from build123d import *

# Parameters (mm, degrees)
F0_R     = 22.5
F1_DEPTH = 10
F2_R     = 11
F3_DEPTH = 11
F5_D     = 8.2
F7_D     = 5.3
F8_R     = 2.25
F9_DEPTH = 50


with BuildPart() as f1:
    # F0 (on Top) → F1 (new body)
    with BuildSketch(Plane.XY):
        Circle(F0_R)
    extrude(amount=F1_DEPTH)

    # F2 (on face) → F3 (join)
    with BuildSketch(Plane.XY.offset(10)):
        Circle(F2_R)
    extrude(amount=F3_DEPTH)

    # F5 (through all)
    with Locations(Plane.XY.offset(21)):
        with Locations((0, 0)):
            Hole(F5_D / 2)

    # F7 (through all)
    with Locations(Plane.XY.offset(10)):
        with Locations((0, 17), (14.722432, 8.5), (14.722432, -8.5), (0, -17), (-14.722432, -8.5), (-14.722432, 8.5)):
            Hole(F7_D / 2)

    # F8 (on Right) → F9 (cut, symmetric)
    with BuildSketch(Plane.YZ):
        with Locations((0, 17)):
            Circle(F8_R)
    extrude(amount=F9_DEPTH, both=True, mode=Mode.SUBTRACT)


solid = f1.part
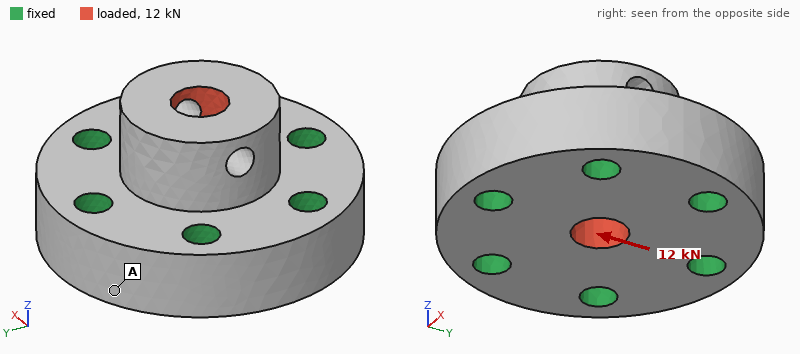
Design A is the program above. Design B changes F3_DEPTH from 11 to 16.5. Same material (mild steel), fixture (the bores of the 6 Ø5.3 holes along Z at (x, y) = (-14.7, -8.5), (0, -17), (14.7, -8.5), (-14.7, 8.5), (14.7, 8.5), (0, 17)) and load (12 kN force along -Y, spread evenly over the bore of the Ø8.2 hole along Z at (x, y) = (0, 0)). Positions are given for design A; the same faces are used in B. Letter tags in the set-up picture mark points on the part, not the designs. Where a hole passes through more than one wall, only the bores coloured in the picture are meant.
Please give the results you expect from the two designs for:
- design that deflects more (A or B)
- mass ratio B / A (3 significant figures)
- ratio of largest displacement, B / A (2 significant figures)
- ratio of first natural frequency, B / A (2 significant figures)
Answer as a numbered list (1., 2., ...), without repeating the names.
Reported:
1. B
2. 1.10
3. 1.8
4. 0.63
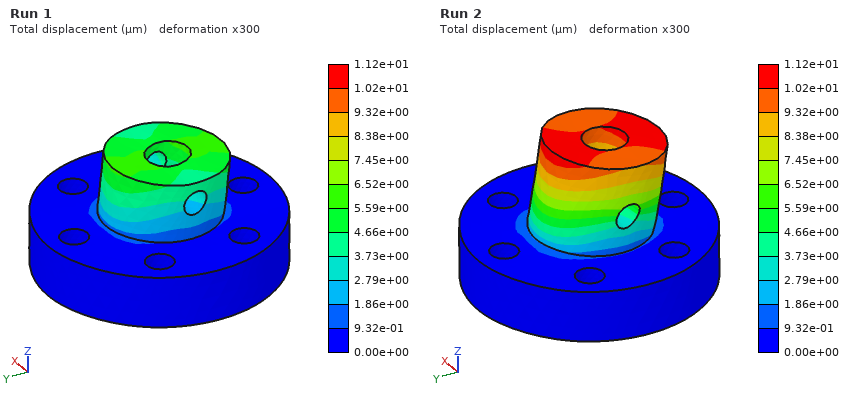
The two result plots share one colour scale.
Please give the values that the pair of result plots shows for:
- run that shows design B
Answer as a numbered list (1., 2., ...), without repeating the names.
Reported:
1. Run 2
